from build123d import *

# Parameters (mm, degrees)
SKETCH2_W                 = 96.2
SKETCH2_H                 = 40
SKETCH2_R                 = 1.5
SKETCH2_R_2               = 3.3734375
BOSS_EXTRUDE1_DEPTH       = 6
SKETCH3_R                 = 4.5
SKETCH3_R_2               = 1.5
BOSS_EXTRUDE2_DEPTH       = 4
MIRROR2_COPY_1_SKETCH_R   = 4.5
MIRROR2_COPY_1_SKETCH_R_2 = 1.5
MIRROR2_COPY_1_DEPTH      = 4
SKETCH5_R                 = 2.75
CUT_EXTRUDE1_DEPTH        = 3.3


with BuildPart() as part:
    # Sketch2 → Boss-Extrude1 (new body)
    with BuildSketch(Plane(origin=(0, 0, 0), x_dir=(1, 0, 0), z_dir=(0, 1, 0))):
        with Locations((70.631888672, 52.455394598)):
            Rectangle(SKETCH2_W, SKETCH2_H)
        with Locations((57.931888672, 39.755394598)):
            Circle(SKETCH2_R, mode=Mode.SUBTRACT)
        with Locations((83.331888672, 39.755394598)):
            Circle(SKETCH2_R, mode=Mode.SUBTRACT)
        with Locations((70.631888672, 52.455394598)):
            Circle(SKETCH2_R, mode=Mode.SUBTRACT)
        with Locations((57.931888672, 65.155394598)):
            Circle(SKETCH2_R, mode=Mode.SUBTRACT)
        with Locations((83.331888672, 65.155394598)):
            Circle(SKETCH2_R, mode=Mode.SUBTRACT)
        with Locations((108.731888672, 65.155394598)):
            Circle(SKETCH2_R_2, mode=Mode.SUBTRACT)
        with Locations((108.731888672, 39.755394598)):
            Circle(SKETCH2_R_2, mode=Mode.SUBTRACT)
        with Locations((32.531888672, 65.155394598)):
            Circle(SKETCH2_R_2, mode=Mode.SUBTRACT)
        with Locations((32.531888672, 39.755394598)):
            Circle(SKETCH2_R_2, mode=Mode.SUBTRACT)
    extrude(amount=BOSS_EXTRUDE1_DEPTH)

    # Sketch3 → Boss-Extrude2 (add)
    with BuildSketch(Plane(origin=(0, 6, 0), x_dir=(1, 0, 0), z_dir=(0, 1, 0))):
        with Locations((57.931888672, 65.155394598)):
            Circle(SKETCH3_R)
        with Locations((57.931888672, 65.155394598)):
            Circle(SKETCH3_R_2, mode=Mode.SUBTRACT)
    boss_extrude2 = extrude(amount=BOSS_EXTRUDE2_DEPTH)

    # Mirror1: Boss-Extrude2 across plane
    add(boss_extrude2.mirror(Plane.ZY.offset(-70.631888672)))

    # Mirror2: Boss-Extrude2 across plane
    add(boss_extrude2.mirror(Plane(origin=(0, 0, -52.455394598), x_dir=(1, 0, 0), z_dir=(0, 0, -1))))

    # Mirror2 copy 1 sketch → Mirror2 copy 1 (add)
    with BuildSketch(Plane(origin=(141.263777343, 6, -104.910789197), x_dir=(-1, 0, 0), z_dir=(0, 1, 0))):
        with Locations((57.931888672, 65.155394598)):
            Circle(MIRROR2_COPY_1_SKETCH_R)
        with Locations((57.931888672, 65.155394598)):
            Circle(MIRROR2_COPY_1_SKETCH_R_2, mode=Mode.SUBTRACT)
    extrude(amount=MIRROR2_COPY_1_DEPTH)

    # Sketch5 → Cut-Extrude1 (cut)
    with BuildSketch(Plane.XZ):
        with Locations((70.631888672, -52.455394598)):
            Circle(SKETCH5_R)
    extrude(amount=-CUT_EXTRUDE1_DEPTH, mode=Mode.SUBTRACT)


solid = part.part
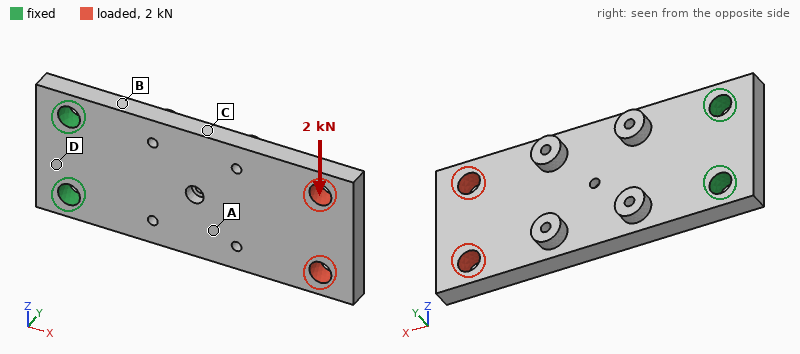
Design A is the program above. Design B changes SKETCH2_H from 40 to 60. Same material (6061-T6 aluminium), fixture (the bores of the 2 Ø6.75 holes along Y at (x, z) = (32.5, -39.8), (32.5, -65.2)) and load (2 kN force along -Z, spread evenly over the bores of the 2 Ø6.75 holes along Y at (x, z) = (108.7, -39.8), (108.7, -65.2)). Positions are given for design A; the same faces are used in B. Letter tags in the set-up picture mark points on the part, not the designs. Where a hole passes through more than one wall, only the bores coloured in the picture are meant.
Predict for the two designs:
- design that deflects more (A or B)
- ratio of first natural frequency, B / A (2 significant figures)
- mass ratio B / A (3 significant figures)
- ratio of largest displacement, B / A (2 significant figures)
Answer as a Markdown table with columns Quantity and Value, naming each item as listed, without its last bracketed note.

| Quantity | Value |
|---|---|
| design that deflects more | A |
| ratio of first natural frequency, B / A | 0.98 |
| mass ratio B / A | 1.50 |
| ratio of largest displacement, B / A | 0.56 |
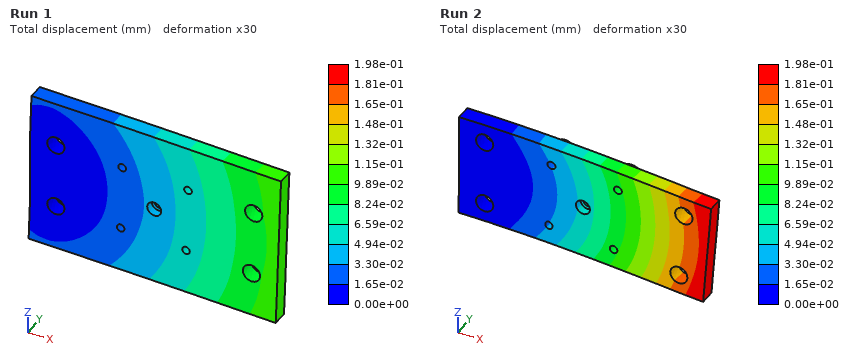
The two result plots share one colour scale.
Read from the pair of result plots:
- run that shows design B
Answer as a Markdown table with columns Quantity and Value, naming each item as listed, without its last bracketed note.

| Quantity | Value |
|---|---|
| run that shows design B | Run 1 |
